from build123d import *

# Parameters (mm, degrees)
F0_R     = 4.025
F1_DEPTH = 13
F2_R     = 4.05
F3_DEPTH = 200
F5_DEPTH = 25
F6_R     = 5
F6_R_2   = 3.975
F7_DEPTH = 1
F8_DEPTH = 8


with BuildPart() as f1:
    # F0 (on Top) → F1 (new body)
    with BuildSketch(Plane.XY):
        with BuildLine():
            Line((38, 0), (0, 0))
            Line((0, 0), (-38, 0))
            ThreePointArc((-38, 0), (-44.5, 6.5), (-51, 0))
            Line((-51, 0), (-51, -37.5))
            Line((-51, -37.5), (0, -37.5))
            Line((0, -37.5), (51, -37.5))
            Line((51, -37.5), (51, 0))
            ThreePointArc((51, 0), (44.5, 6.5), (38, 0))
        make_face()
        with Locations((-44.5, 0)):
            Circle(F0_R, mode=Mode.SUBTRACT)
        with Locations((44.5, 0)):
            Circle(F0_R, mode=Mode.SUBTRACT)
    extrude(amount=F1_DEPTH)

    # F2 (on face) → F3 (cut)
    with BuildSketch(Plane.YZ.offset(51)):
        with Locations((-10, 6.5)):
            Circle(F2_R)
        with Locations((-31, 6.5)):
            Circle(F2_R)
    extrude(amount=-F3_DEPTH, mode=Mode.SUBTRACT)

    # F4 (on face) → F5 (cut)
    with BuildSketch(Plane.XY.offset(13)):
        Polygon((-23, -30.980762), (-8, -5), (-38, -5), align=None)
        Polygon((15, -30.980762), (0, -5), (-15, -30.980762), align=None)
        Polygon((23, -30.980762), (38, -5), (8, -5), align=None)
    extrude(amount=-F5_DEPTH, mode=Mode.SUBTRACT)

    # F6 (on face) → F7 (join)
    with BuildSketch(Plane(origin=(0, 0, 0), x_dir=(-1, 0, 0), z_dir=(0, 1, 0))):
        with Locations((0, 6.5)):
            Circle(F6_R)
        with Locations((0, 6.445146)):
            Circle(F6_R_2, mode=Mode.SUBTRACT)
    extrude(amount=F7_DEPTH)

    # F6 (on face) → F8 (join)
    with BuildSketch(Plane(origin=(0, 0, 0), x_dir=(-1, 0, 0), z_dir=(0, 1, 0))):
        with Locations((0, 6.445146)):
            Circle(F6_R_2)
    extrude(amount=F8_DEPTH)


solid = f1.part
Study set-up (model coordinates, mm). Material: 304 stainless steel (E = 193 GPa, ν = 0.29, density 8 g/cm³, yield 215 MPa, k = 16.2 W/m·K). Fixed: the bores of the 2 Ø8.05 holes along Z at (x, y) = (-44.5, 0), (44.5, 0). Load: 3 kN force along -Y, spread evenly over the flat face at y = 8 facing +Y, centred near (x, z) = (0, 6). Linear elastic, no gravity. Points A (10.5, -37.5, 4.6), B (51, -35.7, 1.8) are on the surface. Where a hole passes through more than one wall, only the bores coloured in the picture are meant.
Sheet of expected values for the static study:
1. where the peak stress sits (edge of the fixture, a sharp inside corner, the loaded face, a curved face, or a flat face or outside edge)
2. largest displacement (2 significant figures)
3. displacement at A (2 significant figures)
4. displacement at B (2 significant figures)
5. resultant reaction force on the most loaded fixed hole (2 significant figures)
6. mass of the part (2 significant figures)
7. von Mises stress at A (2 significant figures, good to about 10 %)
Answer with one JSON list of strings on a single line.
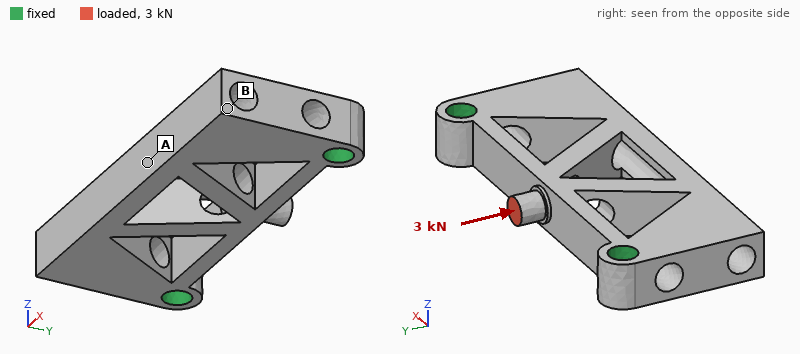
["a curved face", "23 µm", "15 µm", "3.6 µm", "1.8 kN", "230 g", "42 MPa"]
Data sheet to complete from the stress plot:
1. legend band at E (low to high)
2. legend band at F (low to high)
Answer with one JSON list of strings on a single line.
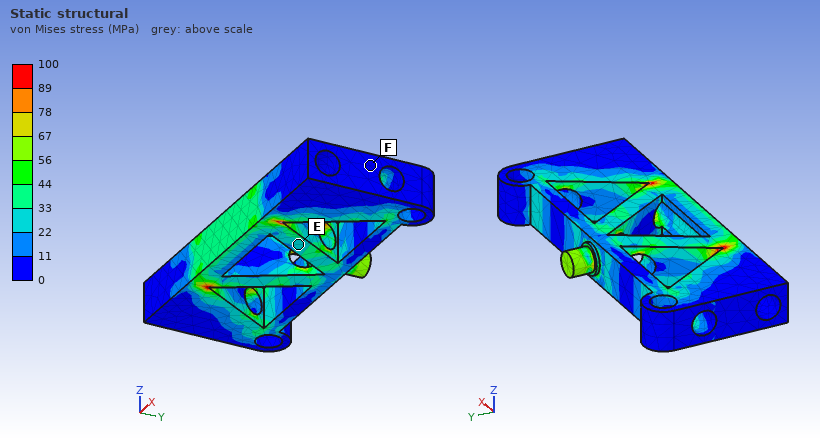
["22 to 33 MPa", "0 to 11 MPa"]
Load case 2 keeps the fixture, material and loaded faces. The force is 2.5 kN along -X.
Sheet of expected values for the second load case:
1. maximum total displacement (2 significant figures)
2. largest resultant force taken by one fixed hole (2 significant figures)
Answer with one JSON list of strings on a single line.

["45 µm", "1.3 kN"]
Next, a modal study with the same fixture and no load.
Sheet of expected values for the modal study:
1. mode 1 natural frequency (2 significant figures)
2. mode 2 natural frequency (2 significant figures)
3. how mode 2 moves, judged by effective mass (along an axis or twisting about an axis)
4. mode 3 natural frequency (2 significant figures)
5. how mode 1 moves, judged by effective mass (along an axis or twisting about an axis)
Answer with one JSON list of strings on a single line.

["3900 Hz", "6300 Hz", "twisting about Y", "6800 Hz", "along Z"]
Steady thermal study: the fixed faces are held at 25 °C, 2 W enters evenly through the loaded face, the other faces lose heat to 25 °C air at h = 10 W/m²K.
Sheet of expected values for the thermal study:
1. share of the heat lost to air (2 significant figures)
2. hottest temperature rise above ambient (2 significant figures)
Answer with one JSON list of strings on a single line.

["39 %", "40 K"]
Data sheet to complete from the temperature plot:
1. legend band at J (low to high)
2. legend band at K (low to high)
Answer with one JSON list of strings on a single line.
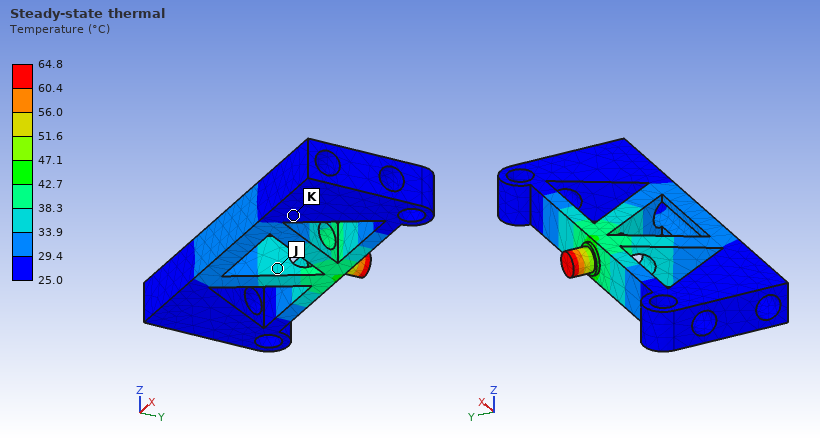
["33.9 to 38.3 °C", "25.0 to 29.4 °C"]
